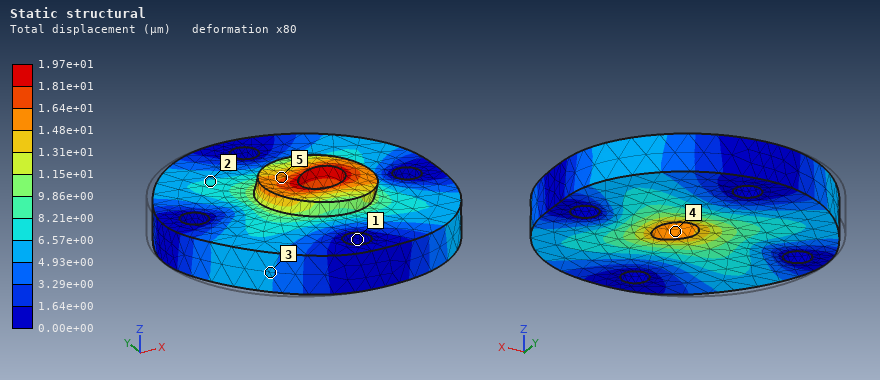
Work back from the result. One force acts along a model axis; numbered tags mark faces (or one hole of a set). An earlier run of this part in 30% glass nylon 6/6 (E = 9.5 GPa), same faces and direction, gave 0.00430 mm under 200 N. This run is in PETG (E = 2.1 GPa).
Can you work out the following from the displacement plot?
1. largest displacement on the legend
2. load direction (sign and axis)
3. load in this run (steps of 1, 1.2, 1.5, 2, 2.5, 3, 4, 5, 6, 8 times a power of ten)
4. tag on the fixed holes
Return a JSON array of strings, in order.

["1.97e+01 µm", "+X", "200 N", "1"]
